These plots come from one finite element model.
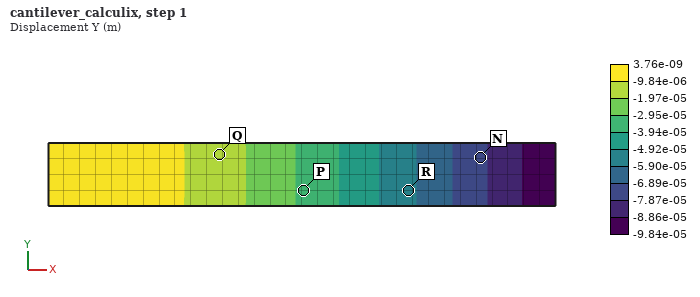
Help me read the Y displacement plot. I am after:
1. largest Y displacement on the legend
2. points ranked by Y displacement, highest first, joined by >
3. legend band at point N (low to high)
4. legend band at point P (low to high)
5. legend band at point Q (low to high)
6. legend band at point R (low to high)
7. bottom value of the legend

3.76e-09 m
Q > P > R > N
-7.87e-05 to -6.89e-05 m
-3.94e-05 to -2.95e-05 m
-1.97e-05 to -9.84e-06 m
-5.90e-05 to -4.92e-05 m
-9.84e-05 m
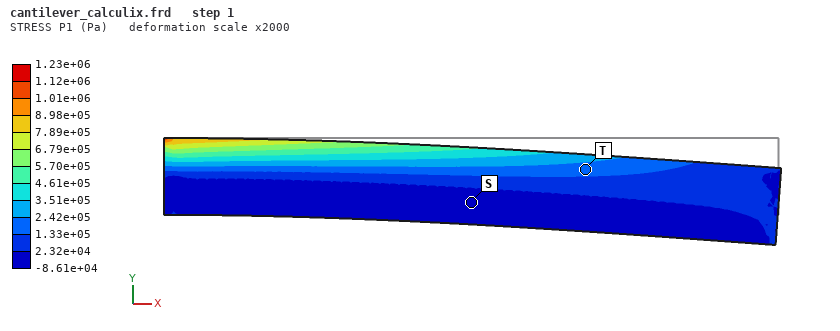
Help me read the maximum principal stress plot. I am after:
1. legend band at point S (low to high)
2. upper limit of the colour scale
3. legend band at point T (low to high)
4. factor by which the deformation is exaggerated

-8.61e+04 to 2.32e+04 Pa
1.23e+06 Pa
1.33e+05 to 2.42e+05 Pa
2000
